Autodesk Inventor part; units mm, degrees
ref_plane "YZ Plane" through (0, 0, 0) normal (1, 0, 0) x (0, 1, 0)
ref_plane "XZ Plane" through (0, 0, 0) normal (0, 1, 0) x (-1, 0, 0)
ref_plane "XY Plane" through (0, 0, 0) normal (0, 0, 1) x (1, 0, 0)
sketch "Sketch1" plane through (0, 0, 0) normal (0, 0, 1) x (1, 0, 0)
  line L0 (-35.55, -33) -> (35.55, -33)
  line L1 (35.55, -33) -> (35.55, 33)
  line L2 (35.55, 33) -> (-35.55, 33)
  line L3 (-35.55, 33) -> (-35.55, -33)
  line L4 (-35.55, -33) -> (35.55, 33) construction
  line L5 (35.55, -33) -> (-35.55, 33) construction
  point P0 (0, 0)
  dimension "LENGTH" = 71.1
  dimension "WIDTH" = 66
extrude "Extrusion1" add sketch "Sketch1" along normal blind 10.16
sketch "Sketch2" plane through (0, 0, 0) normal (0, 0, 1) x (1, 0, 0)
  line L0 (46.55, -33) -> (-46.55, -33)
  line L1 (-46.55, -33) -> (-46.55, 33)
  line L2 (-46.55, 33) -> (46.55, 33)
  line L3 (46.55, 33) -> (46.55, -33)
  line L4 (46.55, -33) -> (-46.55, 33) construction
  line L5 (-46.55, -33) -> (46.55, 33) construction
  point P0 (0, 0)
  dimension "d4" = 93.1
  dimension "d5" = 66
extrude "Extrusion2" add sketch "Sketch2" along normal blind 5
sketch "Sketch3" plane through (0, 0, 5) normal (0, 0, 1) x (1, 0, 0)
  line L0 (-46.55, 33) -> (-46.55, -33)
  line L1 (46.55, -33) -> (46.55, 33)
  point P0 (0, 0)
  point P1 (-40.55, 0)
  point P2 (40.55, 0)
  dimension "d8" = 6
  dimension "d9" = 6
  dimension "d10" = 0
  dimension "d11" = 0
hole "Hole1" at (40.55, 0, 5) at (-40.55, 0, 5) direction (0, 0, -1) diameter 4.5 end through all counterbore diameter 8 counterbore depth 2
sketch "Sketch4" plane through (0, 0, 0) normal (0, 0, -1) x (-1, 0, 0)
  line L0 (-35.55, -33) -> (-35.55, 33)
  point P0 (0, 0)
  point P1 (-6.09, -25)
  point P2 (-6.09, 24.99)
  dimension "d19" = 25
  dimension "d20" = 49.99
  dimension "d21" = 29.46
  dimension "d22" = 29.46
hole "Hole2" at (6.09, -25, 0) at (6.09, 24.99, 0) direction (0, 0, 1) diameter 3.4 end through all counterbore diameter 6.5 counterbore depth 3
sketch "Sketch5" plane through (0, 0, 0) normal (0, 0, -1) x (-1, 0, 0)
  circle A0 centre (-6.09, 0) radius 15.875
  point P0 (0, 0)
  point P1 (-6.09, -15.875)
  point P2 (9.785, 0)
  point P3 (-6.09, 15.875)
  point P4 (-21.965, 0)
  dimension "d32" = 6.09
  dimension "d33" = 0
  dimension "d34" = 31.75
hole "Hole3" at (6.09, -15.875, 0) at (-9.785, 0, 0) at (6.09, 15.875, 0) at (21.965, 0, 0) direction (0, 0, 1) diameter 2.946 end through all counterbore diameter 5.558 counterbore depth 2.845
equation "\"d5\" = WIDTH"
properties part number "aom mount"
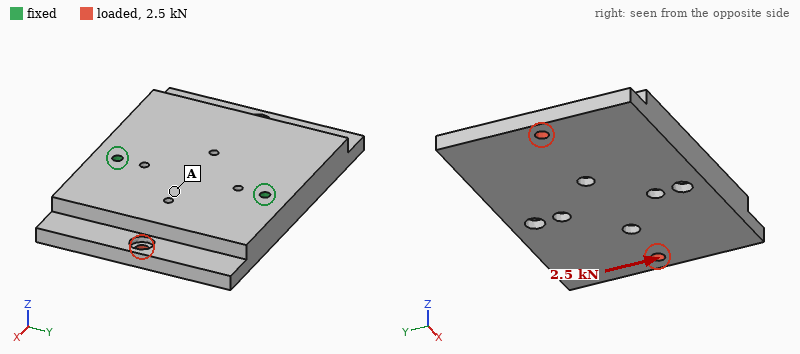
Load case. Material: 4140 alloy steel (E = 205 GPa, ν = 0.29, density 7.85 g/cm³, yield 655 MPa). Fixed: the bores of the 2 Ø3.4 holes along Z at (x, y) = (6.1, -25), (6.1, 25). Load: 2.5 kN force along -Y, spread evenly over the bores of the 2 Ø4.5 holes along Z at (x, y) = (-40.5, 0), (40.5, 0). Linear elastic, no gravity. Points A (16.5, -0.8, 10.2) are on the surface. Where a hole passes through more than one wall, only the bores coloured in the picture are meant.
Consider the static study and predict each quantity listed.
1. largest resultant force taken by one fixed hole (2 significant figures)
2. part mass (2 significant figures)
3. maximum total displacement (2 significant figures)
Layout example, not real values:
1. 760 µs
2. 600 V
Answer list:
1. 1.3 kN
2. 420 g
3. 4.1 µm
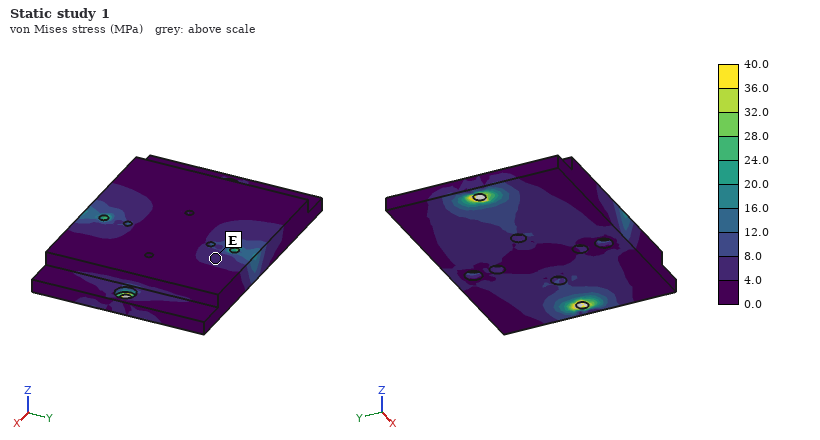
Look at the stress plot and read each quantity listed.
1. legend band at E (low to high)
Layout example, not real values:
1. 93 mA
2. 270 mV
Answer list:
1. 4.0 to 8.0 MPa
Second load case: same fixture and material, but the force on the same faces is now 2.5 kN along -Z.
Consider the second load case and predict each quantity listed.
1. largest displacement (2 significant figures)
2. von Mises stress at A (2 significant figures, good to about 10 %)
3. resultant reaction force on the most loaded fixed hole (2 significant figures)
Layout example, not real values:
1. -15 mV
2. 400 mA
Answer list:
1. 74 µm
2. 31 MPa
3. 1.3 kN
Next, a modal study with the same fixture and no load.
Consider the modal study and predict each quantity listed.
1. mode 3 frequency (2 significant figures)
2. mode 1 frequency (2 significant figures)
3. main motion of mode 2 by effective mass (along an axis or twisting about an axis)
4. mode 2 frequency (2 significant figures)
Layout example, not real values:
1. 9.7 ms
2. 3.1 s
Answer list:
1. 5600 Hz
2. 2100 Hz
3. along Z
4. 4500 Hz
